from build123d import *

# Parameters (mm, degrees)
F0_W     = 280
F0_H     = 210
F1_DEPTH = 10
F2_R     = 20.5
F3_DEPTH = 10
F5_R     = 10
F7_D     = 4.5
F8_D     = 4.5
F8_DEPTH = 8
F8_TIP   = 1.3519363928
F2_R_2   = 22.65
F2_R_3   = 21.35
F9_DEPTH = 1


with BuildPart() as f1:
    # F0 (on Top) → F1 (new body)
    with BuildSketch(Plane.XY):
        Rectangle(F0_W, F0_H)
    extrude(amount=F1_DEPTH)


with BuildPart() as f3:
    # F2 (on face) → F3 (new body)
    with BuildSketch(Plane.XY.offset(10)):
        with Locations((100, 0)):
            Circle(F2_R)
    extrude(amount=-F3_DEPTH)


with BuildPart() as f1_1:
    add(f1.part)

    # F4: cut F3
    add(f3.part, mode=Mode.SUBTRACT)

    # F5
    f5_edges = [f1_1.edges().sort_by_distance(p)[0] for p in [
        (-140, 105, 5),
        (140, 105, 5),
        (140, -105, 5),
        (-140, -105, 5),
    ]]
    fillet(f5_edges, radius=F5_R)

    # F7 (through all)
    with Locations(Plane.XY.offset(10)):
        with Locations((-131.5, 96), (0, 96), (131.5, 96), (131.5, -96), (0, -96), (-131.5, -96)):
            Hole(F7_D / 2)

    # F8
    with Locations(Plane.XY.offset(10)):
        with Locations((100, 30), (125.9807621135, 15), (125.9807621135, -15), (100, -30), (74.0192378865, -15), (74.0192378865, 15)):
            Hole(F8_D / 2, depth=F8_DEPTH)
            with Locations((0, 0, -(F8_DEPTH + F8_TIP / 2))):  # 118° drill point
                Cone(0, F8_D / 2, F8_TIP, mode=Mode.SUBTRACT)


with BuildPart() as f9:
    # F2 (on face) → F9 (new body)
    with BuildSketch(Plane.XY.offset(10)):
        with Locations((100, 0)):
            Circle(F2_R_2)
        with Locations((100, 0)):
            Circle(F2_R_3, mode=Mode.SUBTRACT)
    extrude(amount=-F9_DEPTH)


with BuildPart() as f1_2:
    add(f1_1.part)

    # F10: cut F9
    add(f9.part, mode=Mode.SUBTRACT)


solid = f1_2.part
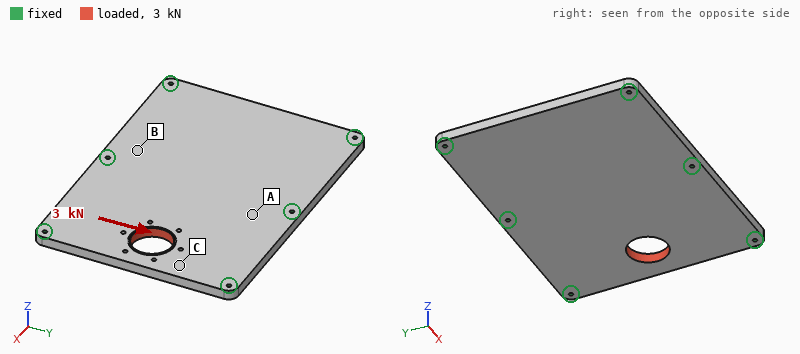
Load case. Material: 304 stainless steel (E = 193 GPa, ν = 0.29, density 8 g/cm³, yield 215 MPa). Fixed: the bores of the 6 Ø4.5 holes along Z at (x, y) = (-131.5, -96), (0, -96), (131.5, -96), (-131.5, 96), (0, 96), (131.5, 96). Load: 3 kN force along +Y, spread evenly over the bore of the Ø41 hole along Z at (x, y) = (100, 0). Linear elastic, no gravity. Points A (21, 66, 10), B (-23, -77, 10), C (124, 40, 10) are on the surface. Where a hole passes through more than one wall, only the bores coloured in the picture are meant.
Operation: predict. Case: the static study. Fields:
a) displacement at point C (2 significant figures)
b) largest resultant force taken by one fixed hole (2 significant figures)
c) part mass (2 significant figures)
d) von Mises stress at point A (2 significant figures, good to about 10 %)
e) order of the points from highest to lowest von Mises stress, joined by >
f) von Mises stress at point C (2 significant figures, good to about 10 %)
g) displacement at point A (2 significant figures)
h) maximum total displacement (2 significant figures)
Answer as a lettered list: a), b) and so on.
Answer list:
a) 1.0 µm
b) 930 N
c) 4.6 kg
d) 1.4 MPa
e) C > A > B
f) 2.2 MPa
g) 0.42 µm
h) 1.5 µm
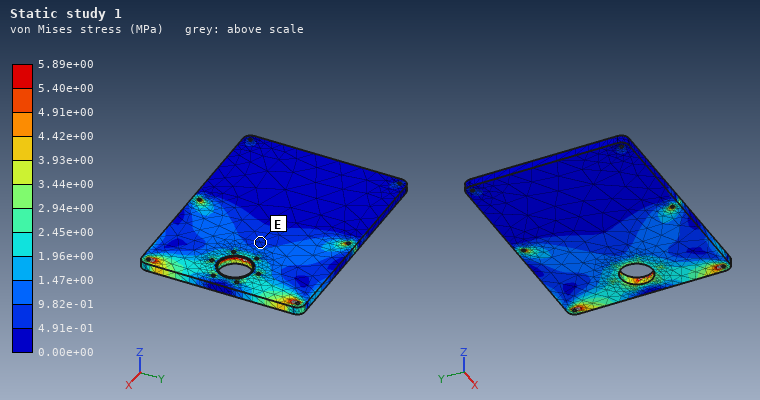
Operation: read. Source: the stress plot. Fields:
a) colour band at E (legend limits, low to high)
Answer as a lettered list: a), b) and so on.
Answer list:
a) 4.91e-01 to 9.82e-01 MPa
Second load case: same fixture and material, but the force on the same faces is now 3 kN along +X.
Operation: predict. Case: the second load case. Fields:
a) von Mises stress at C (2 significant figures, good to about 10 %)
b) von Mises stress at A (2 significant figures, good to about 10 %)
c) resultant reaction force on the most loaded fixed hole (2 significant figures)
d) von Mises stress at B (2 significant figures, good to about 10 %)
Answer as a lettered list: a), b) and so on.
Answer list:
a) 1.3 MPa
b) 1.5 MPa
c) 800 N
d) 0.85 MPa
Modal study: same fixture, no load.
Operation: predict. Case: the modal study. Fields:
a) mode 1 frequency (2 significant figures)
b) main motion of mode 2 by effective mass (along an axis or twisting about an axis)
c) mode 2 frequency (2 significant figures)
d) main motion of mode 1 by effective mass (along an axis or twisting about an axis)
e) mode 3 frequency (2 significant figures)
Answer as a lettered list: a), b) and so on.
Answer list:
a) 930 Hz
b) twisting about Y
c) 1100 Hz
d) along Z
e) 1800 Hz
